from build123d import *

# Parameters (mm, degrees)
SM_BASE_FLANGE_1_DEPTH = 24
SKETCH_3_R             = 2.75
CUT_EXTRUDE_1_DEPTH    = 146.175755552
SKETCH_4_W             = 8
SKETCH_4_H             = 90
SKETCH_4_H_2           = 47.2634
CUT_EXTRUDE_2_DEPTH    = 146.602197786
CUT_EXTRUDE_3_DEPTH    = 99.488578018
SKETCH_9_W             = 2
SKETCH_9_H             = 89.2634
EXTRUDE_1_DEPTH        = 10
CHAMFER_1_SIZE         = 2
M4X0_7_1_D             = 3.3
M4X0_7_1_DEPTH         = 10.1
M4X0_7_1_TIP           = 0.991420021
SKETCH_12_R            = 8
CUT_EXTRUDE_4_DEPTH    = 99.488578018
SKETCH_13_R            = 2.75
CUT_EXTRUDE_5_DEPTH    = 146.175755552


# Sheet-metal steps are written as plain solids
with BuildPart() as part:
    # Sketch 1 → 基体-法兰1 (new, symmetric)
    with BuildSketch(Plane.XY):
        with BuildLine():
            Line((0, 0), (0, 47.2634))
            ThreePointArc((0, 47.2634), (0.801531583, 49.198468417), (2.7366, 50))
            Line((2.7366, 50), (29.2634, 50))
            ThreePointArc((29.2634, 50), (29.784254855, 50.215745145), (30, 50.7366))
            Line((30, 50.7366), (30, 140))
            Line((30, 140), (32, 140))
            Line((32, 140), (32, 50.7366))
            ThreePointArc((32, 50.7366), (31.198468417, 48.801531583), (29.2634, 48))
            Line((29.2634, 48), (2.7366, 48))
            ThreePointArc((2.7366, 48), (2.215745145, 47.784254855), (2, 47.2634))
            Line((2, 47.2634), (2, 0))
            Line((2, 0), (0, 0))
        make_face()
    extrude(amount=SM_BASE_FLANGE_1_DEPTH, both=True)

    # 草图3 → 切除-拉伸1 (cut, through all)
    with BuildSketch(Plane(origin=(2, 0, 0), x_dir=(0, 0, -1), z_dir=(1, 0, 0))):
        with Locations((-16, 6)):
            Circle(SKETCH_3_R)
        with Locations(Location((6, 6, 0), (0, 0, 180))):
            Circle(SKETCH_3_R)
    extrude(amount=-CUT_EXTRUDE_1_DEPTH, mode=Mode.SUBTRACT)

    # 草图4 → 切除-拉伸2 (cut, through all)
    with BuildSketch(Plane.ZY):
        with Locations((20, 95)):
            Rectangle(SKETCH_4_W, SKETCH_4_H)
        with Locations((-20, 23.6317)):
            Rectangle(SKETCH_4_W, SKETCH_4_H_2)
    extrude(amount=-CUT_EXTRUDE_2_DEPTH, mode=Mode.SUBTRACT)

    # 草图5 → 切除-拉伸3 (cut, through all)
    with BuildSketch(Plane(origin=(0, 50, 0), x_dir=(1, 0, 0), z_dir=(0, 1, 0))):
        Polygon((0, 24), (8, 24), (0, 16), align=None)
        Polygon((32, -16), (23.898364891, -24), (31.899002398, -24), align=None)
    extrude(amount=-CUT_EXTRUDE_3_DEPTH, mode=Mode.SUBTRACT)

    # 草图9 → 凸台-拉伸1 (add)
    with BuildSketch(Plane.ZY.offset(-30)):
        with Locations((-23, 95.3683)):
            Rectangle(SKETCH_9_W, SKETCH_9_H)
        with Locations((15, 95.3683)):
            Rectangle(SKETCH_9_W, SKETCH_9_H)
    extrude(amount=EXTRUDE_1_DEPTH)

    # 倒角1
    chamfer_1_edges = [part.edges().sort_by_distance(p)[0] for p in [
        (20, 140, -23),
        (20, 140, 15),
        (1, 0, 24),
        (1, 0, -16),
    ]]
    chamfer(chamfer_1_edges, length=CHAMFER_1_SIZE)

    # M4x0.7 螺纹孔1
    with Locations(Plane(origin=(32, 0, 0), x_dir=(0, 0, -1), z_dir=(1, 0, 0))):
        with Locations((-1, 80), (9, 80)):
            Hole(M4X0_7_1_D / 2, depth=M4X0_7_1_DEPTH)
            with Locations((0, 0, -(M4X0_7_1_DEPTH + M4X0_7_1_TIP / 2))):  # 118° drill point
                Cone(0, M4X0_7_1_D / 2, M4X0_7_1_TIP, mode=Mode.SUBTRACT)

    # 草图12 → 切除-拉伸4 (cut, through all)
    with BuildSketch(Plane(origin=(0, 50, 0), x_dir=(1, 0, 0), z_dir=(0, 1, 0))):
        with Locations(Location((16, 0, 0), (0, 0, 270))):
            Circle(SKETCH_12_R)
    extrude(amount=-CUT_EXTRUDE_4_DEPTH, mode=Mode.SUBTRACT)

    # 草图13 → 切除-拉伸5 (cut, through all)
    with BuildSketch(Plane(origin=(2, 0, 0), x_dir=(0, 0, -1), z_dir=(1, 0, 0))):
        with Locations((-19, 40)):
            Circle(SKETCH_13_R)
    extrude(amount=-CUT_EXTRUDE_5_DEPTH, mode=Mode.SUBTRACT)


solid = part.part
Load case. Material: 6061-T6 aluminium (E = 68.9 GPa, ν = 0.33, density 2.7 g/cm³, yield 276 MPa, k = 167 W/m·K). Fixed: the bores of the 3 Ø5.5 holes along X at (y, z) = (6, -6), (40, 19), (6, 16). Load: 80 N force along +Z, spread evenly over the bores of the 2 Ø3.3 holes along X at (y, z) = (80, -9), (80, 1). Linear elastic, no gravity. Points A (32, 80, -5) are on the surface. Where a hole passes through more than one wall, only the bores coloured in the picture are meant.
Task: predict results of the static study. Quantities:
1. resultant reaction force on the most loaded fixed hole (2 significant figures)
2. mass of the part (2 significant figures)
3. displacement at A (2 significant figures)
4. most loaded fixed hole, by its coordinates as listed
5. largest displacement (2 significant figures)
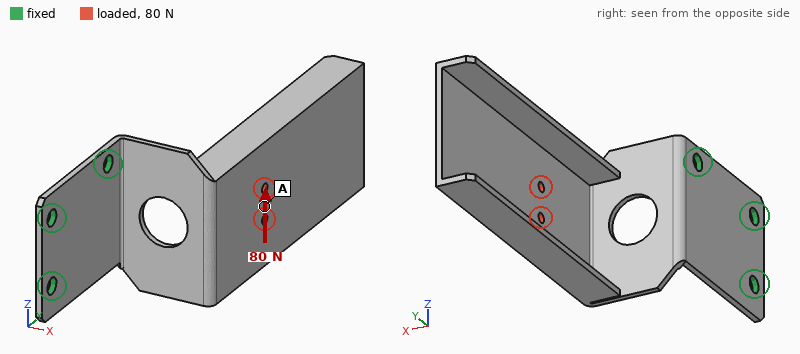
140 N
45 g
0.66 mm
(40, 19)
1.6 mm
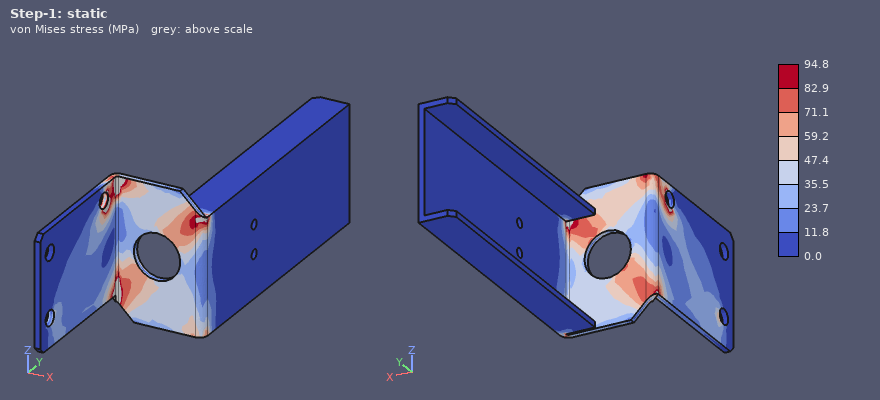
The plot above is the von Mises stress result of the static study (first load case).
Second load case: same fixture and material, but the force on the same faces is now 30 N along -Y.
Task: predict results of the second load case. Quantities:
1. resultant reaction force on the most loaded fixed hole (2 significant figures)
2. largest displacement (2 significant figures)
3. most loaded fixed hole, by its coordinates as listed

21 N
1.4 mm
(6, -6)
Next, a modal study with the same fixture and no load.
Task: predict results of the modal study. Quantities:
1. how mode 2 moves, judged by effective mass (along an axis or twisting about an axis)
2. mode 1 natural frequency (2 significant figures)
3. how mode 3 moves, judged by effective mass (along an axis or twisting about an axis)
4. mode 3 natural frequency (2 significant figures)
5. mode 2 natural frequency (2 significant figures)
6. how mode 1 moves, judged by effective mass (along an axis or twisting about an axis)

along Z
98 Hz
along Y
520 Hz
200 Hz
along X
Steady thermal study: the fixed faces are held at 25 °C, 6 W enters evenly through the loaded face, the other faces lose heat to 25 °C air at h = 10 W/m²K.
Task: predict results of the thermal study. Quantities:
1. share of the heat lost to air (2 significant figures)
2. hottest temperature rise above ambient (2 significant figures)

41 %
24 K
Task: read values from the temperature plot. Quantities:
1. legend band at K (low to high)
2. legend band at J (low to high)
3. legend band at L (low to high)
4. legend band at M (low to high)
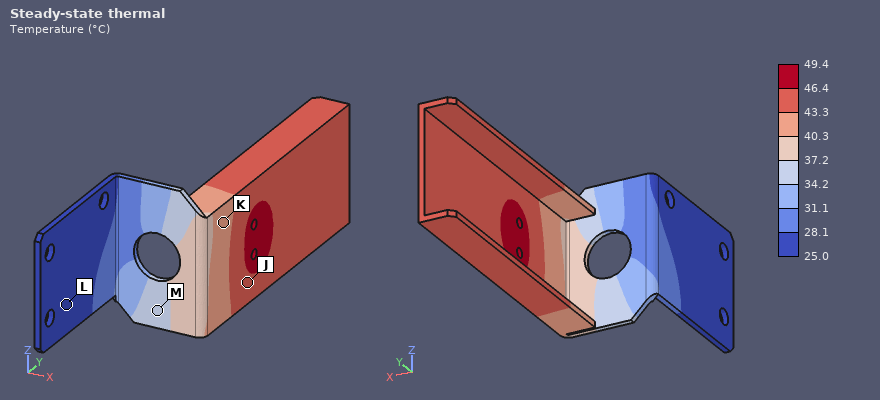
40.3 to 43.3 °C
43.3 to 46.4 °C
25.0 to 28.1 °C
34.2 to 37.2 °C
